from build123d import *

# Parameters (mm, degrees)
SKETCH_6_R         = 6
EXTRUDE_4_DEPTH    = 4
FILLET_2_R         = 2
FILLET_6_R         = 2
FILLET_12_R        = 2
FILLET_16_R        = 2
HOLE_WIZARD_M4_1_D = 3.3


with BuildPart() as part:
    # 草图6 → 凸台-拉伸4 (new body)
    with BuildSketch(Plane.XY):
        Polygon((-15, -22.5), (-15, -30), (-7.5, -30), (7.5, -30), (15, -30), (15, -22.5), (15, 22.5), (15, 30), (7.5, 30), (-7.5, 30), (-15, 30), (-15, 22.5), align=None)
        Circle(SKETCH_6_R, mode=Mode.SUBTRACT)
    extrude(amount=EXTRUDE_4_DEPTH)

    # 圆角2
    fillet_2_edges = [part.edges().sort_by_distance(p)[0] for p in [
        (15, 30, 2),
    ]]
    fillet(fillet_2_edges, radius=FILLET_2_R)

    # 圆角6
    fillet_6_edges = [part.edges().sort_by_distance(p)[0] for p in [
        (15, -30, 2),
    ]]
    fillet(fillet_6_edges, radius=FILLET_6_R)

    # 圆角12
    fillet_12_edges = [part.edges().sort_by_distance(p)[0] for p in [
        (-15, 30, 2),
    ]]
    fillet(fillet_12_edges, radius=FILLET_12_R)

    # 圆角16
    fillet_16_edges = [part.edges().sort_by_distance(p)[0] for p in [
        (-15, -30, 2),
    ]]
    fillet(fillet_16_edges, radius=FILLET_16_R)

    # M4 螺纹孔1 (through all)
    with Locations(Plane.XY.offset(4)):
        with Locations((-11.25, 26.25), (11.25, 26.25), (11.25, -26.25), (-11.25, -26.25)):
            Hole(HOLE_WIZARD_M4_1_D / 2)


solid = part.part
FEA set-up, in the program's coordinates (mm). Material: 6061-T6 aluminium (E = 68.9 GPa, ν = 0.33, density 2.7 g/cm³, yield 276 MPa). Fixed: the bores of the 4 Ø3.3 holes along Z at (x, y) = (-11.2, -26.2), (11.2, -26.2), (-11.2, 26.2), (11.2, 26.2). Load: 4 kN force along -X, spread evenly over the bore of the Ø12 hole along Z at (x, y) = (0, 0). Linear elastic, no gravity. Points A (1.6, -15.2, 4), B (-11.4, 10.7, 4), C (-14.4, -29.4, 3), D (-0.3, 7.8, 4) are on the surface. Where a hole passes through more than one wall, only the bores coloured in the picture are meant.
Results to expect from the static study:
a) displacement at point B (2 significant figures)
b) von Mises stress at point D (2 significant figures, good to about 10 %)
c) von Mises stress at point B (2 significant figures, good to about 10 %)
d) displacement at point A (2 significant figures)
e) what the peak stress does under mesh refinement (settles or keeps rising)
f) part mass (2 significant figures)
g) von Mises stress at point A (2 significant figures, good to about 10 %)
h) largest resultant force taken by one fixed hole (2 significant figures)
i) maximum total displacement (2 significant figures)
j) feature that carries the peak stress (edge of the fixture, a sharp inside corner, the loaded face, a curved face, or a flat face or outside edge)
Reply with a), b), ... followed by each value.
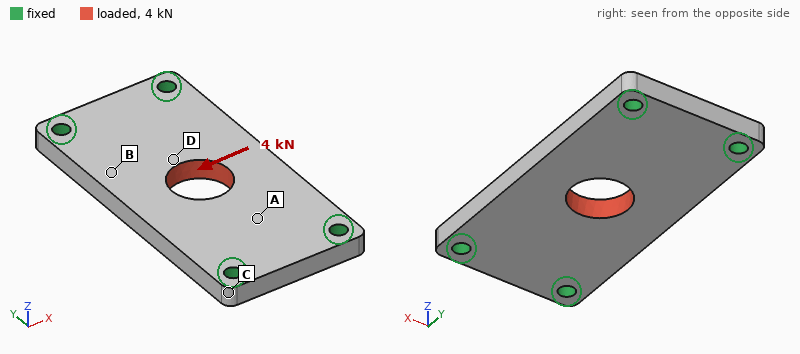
a) 15 µm
b) 49 MPa
c) 21 MPa
d) 10 µm
e) keeps rising
f) 18 g
g) 42 MPa
h) 1.5 kN
i) 24 µm
j) edge of the fixture
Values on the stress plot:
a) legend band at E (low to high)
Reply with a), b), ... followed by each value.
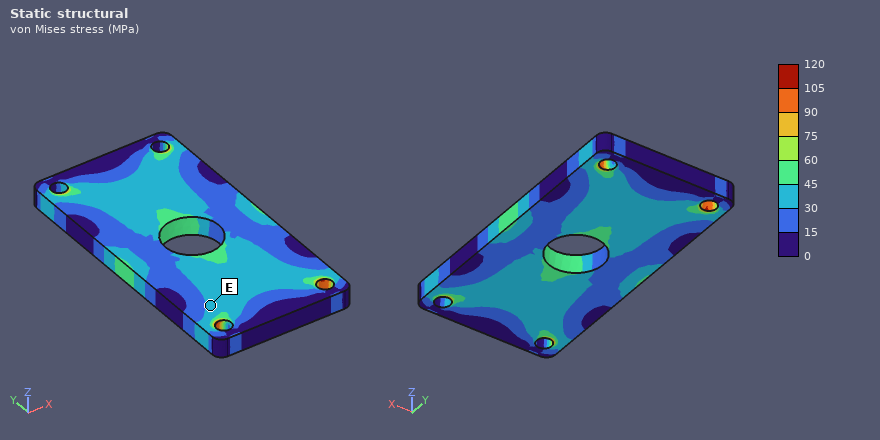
a) 30 to 45 MPa
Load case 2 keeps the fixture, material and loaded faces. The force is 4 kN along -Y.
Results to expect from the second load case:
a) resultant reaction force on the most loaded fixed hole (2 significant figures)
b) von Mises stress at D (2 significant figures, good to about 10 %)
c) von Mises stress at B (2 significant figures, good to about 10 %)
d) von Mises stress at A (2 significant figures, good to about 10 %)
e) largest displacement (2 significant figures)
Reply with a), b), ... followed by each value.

a) 1.0 kN
b) 26 MPa
c) 14 MPa
d) 17 MPa
e) 8.5 µm
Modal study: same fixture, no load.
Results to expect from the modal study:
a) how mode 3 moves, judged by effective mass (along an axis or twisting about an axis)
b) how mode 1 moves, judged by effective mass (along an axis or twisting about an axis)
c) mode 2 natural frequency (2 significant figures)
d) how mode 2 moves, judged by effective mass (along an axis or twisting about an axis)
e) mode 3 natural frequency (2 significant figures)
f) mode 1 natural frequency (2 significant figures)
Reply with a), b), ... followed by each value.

a) twisting about X
b) along Z
c) 11 kHz
d) twisting about Y
e) 18 kHz
f) 7100 Hz
